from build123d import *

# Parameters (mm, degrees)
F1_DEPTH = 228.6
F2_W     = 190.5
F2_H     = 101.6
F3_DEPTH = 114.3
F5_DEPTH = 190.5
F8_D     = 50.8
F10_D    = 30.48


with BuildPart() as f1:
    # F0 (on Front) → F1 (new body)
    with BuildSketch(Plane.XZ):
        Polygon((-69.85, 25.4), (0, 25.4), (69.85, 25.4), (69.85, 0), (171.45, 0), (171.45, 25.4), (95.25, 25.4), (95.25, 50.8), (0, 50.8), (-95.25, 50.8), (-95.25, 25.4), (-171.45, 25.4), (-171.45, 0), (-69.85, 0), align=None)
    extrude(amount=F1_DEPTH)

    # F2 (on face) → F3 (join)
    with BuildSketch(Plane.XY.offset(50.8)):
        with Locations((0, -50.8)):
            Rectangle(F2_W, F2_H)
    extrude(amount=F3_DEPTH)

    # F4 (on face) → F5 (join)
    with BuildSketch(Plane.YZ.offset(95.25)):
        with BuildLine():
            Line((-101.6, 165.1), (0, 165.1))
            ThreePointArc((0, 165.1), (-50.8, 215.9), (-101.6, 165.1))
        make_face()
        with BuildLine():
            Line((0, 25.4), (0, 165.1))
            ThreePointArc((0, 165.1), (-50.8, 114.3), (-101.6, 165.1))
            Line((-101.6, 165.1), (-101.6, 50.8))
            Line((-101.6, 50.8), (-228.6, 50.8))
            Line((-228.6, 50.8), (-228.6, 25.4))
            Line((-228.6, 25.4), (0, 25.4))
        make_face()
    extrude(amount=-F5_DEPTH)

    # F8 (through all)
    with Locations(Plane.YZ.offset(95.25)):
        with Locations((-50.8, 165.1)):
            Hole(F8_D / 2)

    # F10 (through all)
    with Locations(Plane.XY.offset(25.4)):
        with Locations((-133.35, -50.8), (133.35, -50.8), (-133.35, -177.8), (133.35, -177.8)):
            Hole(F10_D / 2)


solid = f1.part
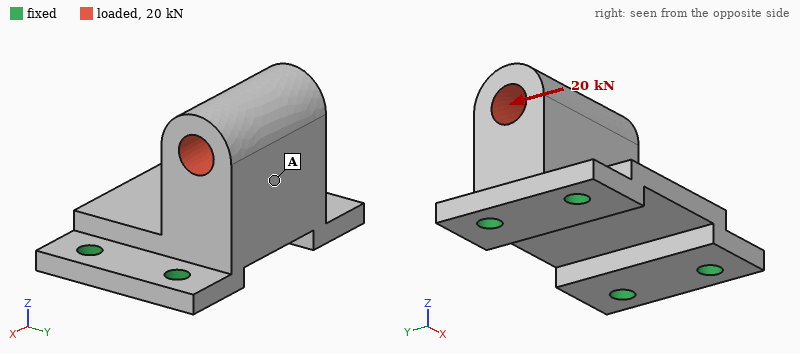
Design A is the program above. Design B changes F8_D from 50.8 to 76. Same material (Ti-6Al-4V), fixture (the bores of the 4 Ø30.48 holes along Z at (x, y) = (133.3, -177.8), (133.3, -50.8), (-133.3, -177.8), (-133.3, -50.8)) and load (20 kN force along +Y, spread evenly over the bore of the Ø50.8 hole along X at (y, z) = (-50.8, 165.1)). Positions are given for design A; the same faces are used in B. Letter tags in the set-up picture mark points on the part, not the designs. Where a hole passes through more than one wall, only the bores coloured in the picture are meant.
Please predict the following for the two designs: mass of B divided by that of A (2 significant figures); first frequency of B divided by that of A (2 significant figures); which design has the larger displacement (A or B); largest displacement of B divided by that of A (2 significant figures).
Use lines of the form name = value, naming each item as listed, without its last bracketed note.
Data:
mass of B divided by that of A = 0.90
first frequency of B divided by that of A = 1.2
which design has the larger displacement = B
largest displacement of B divided by that of A = 1.2
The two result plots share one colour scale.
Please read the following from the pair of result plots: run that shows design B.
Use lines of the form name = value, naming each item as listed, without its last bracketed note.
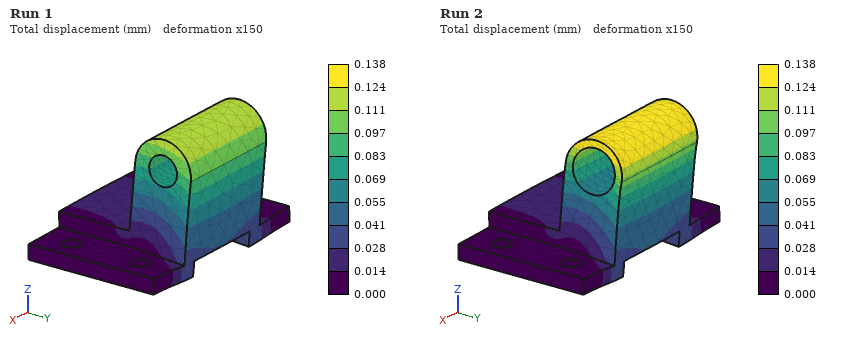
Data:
run that shows design B = Run 2
